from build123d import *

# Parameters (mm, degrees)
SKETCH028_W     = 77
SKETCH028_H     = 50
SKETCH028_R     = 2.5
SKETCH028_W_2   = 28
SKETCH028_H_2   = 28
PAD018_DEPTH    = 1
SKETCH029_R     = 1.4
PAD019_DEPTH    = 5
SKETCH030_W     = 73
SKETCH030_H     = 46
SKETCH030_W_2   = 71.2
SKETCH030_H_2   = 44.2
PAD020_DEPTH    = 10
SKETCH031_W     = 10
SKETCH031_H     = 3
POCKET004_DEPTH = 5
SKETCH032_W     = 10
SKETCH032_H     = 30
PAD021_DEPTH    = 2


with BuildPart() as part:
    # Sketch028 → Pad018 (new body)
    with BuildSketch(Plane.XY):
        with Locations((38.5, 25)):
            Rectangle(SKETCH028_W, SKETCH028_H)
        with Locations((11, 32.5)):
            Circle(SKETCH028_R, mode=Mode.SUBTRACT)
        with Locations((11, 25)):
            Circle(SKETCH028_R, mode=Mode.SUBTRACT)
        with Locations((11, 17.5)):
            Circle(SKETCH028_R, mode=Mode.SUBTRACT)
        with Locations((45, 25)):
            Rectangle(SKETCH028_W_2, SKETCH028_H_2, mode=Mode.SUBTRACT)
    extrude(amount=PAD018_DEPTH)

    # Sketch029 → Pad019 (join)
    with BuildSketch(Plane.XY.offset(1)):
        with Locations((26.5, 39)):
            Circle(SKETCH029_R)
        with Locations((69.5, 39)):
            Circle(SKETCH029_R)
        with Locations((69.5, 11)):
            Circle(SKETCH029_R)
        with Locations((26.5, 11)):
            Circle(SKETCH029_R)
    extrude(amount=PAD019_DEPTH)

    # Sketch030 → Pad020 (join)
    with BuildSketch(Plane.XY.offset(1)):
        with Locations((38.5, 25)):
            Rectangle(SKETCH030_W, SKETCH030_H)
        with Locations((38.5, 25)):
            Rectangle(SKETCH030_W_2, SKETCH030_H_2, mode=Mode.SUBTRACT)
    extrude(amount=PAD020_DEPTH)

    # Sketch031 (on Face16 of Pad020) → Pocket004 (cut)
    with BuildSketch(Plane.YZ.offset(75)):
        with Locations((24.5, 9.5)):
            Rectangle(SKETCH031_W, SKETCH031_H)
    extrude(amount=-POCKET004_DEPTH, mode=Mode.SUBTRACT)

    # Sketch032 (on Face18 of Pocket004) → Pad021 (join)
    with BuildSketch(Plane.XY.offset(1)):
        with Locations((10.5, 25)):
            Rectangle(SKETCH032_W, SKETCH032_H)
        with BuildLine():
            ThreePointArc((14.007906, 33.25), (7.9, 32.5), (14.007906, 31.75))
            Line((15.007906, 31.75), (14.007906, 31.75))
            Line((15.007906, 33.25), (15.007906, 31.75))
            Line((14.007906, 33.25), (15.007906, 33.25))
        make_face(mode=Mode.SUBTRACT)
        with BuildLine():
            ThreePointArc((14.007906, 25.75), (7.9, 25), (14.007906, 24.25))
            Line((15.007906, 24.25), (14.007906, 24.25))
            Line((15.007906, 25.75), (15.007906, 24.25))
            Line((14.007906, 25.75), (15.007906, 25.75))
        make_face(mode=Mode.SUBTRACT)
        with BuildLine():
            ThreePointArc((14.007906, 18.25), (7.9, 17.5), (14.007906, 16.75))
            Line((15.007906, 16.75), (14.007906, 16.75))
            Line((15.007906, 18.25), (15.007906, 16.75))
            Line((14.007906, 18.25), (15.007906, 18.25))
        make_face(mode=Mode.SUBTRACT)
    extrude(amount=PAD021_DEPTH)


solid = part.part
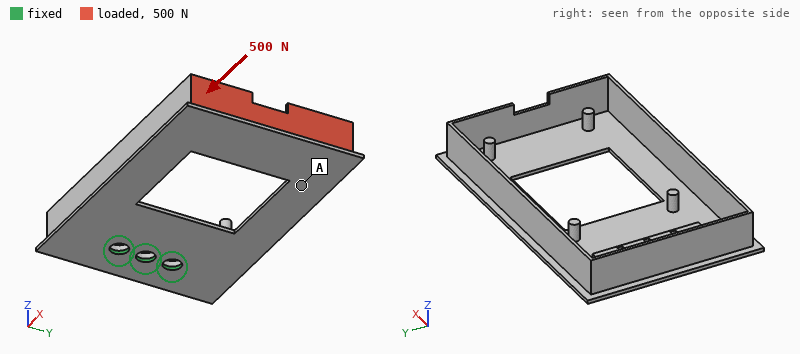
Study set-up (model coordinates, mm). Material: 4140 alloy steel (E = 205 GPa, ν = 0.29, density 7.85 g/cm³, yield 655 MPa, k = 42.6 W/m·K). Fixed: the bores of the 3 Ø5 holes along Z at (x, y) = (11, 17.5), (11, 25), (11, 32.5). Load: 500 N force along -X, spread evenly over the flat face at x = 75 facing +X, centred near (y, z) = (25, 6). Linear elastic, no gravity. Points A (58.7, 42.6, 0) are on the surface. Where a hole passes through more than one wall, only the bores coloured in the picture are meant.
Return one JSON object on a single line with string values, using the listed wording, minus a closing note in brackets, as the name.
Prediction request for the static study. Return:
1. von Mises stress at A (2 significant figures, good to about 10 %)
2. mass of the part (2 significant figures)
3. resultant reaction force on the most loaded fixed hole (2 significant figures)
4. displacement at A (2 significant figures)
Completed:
{"von Mises stress at A": "22 MPa", "mass of the part": "44 g", "resultant reaction force on the most loaded fixed hole": "260 N", "displacement at A": "0.28 mm"}
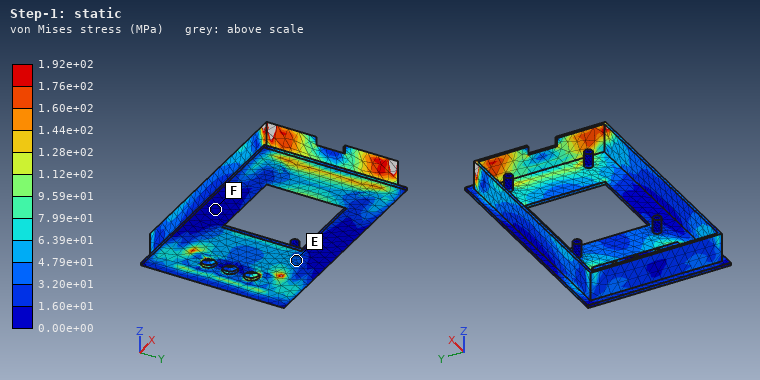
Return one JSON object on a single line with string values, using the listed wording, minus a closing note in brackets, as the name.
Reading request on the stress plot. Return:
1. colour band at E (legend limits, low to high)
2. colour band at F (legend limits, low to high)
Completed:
{"colour band at E": "3.20e+01 to 4.79e+01 MPa", "colour band at F": "0.00e+00 to 1.60e+01 MPa"}
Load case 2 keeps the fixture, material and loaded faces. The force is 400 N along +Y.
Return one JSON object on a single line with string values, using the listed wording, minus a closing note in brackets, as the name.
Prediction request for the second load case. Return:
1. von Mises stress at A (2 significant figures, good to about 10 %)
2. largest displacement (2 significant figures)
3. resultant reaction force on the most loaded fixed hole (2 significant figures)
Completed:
{"von Mises stress at A": "63 MPa", "largest displacement": "1.1 mm", "resultant reaction force on the most loaded fixed hole": "1.3 kN"}
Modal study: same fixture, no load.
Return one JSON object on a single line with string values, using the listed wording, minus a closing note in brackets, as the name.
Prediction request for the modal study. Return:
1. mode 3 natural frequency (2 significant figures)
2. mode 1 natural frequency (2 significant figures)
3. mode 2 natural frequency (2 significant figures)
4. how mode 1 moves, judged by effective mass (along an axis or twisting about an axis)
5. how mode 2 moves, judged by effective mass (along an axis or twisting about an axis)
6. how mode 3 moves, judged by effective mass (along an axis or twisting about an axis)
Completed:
{"mode 3 natural frequency": "2600 Hz", "mode 1 natural frequency": "420 Hz", "mode 2 natural frequency": "560 Hz", "how mode 1 moves, judged by effective mass": "along Z", "how mode 2 moves, judged by effective mass": "twisting about X", "how mode 3 moves, judged by effective mass": "along Y"}
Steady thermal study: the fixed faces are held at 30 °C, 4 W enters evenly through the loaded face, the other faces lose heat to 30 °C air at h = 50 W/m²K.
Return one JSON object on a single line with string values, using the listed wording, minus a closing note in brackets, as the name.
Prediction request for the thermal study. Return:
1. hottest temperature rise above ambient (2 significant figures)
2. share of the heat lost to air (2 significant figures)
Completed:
{"hottest temperature rise above ambient": "33 K", "share of the heat lost to air": "97 %"}
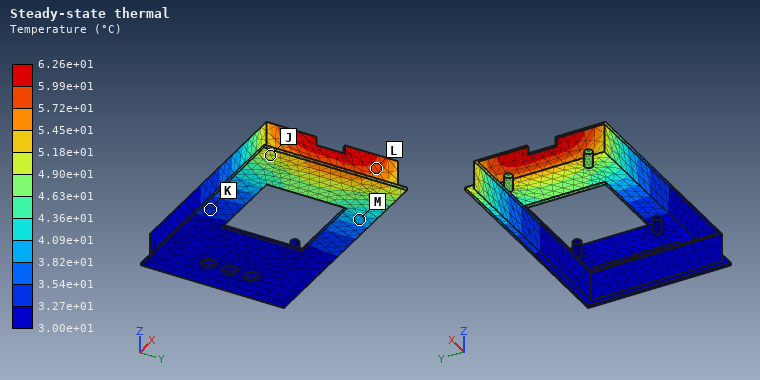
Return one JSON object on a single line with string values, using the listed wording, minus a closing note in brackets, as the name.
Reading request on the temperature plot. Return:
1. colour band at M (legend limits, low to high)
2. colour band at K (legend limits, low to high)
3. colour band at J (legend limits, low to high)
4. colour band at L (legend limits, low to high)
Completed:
{"colour band at M": "3.82e+01 to 4.09e+01 °C", "colour band at K": "3.27e+01 to 3.54e+01 °C", "colour band at J": "4.90e+01 to 5.18e+01 °C", "colour band at L": "5.72e+01 to 5.99e+01 °C"}
